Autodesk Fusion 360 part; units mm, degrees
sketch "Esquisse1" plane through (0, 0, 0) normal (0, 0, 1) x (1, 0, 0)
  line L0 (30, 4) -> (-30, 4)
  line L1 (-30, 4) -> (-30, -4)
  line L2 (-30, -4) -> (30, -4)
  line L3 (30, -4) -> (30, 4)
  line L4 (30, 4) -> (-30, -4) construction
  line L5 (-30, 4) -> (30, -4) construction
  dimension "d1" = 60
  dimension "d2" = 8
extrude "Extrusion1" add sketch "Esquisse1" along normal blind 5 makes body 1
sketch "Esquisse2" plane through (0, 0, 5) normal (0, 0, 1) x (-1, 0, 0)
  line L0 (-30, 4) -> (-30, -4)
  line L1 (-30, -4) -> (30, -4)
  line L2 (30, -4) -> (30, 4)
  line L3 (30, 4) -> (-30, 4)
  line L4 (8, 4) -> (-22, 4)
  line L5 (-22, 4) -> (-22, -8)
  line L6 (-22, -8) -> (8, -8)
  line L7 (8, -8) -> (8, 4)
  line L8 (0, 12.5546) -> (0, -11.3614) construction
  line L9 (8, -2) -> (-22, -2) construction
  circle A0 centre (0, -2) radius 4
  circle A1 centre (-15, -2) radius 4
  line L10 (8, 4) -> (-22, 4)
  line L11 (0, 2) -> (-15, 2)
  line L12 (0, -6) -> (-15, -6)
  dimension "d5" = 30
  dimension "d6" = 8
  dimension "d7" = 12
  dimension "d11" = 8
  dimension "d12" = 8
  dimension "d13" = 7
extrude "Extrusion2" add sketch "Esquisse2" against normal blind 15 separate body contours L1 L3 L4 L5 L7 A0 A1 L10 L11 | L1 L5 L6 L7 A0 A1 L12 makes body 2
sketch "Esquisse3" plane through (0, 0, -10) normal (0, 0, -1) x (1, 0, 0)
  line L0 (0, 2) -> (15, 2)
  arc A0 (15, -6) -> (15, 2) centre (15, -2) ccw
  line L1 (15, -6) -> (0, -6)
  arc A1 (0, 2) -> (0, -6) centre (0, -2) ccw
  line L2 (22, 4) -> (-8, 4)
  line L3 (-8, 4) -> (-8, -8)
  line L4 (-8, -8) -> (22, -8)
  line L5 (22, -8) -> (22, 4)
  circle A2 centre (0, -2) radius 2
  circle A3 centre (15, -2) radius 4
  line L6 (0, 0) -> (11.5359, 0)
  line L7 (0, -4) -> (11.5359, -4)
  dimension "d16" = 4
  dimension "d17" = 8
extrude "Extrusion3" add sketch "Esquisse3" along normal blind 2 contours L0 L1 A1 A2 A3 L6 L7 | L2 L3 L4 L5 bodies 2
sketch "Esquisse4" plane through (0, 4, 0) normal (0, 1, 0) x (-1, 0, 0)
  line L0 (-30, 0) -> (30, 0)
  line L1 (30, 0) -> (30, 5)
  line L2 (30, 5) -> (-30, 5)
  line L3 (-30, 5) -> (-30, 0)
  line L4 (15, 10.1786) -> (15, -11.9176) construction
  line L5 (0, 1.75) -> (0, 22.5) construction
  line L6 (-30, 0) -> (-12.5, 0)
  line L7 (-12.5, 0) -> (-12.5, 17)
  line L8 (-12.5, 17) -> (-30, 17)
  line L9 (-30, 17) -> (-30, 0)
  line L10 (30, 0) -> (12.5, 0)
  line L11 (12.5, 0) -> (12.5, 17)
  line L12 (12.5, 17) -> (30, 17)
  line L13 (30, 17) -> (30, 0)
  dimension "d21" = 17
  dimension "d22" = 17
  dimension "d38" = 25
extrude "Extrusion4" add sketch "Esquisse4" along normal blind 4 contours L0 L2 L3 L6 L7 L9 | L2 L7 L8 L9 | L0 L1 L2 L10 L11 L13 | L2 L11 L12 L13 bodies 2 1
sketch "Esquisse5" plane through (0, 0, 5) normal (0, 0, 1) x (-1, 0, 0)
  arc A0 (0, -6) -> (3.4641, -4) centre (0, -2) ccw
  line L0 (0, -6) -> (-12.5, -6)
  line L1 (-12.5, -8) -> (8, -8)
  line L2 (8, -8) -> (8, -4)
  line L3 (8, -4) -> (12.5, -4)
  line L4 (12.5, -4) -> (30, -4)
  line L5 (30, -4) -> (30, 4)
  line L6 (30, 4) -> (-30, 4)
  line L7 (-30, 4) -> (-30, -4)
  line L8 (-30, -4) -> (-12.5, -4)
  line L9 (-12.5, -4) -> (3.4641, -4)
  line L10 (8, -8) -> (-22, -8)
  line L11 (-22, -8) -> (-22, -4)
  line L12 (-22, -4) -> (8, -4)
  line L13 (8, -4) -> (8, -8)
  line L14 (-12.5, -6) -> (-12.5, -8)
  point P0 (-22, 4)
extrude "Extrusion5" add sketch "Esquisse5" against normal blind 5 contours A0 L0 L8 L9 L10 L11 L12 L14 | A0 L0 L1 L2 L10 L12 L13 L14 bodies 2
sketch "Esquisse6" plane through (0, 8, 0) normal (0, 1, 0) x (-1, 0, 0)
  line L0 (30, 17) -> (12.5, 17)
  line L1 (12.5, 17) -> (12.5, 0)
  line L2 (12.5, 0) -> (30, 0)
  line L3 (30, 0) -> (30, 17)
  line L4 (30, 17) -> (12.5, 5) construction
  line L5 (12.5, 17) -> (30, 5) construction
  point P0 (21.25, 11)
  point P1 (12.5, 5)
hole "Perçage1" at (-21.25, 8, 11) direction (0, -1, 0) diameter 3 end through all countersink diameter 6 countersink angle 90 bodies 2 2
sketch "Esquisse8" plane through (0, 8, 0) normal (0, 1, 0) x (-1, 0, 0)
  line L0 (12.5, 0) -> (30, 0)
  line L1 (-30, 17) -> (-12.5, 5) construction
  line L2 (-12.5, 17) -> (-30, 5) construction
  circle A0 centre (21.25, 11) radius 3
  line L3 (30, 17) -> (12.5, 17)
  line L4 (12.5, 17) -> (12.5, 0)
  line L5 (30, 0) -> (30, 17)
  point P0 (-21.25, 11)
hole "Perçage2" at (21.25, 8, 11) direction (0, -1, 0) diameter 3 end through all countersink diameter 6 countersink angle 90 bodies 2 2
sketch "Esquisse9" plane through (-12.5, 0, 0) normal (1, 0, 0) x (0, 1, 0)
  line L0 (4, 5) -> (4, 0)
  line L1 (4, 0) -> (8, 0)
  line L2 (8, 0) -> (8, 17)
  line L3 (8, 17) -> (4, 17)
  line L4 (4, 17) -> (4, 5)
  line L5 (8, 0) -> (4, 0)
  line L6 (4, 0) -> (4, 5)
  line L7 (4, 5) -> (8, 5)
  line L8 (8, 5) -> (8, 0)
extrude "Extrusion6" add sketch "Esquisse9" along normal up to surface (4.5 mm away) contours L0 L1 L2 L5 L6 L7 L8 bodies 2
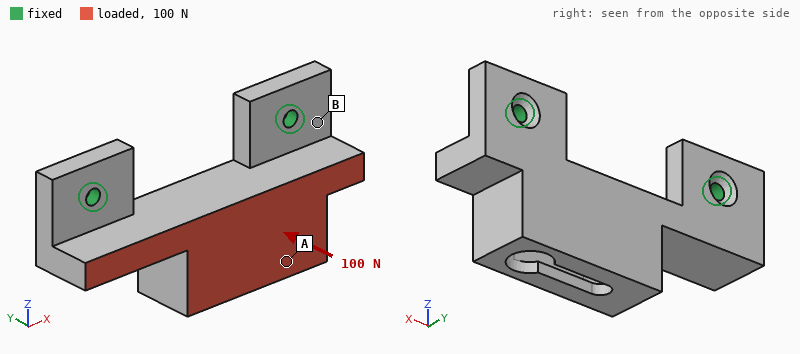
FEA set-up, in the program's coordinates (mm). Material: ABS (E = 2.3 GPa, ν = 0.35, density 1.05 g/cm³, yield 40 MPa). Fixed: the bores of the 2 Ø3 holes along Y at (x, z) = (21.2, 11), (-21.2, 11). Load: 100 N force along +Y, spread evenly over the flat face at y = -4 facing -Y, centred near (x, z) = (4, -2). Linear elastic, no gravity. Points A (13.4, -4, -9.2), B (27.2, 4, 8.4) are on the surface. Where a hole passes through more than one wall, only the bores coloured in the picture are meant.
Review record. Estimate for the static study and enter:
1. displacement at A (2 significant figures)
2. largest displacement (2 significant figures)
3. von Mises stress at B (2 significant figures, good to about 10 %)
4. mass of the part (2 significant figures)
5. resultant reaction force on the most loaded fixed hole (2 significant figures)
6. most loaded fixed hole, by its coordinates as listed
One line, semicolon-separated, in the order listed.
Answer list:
0.69 mm; 0.78 mm; 9.2 MPa; 8.0 g; 59 N; (21.2, 11)
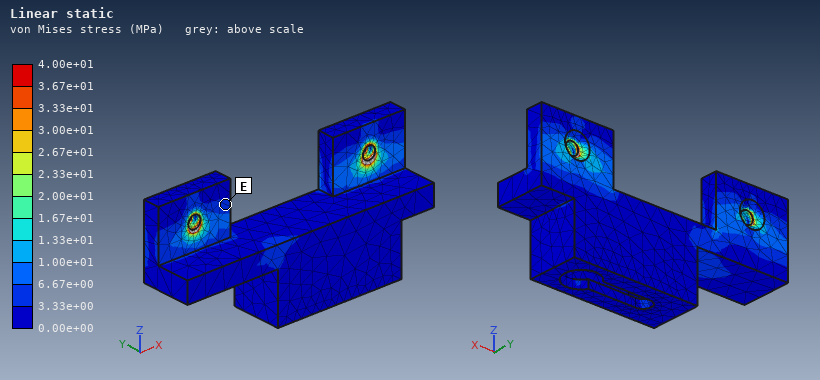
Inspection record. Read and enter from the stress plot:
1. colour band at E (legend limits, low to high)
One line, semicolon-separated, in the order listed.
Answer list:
3.33e+00 to 6.67e+00 MPa
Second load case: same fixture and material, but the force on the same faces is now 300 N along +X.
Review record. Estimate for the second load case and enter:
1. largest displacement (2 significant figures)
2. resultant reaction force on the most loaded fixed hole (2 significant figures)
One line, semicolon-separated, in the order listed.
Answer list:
0.17 mm; 180 N
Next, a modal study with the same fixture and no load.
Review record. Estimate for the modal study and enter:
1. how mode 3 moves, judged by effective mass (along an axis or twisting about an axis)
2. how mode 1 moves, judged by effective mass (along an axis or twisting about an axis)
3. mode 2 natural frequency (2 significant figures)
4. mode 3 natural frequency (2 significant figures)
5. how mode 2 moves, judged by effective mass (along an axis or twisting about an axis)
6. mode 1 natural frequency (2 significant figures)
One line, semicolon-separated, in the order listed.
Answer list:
along X; along Y; 2800 Hz; 3900 Hz; twisting about Z; 950 Hz
